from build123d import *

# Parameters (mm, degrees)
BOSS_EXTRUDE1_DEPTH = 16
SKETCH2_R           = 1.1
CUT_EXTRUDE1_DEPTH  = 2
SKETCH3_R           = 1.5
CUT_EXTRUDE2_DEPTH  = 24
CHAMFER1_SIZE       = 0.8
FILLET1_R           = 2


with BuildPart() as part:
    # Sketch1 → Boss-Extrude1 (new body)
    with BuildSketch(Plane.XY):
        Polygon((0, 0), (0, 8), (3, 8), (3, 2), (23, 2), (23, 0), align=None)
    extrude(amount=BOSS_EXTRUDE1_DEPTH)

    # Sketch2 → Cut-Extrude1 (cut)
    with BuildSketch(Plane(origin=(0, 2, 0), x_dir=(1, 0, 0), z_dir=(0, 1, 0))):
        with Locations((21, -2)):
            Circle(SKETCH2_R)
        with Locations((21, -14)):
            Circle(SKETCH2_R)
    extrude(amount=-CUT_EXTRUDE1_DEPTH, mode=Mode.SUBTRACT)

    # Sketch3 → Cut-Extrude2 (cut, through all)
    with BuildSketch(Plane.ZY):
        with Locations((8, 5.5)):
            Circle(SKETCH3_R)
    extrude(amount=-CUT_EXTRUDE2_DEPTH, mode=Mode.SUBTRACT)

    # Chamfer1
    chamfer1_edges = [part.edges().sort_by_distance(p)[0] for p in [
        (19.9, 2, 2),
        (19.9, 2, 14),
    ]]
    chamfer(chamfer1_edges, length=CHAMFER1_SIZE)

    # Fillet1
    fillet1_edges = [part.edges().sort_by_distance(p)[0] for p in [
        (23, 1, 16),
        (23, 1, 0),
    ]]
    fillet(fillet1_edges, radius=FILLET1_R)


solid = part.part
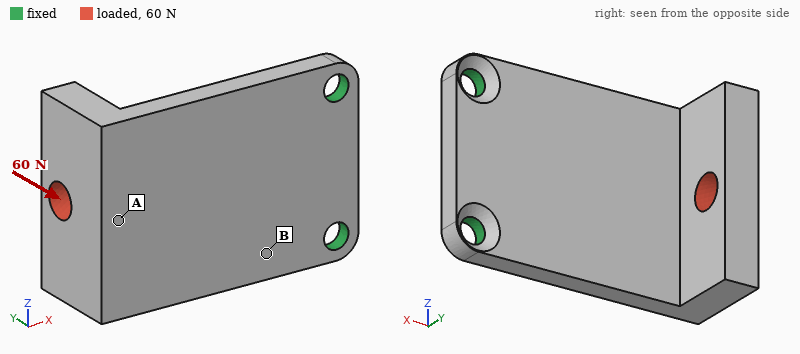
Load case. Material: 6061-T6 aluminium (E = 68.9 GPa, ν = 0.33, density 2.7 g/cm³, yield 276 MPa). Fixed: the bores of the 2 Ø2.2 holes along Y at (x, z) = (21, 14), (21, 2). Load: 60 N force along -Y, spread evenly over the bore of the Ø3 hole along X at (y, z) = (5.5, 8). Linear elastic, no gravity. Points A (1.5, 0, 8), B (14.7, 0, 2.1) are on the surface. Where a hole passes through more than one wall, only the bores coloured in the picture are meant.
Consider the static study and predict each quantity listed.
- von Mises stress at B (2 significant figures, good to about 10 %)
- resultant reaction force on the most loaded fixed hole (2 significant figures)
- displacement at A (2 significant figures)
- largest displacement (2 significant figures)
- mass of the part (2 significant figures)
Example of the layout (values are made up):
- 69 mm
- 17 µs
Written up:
- 75 MPa
- 31 N
- 0.25 mm
- 0.31 mm
- 2.6 g
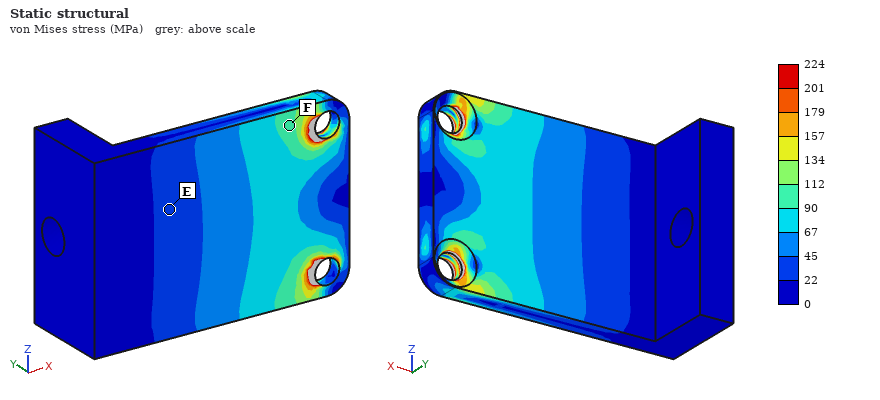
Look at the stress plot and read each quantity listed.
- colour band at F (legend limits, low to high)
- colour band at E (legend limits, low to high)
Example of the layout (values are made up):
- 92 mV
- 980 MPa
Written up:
- 90 to 112 MPa
- 22 to 45 MPa
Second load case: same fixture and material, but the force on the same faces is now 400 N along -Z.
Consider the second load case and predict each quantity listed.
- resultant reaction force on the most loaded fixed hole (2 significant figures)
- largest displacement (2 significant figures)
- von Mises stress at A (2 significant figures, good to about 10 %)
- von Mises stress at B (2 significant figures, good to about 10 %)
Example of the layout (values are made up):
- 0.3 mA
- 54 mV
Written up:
- 670 N
- 0.25 mm
- 44 MPa
- 130 MPa
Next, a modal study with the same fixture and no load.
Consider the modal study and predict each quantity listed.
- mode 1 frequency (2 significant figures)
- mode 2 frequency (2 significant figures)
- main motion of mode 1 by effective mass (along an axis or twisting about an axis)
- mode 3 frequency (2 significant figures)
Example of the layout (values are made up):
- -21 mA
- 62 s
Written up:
- 2100 Hz
- 6600 Hz
- along Y
- 13 kHz
